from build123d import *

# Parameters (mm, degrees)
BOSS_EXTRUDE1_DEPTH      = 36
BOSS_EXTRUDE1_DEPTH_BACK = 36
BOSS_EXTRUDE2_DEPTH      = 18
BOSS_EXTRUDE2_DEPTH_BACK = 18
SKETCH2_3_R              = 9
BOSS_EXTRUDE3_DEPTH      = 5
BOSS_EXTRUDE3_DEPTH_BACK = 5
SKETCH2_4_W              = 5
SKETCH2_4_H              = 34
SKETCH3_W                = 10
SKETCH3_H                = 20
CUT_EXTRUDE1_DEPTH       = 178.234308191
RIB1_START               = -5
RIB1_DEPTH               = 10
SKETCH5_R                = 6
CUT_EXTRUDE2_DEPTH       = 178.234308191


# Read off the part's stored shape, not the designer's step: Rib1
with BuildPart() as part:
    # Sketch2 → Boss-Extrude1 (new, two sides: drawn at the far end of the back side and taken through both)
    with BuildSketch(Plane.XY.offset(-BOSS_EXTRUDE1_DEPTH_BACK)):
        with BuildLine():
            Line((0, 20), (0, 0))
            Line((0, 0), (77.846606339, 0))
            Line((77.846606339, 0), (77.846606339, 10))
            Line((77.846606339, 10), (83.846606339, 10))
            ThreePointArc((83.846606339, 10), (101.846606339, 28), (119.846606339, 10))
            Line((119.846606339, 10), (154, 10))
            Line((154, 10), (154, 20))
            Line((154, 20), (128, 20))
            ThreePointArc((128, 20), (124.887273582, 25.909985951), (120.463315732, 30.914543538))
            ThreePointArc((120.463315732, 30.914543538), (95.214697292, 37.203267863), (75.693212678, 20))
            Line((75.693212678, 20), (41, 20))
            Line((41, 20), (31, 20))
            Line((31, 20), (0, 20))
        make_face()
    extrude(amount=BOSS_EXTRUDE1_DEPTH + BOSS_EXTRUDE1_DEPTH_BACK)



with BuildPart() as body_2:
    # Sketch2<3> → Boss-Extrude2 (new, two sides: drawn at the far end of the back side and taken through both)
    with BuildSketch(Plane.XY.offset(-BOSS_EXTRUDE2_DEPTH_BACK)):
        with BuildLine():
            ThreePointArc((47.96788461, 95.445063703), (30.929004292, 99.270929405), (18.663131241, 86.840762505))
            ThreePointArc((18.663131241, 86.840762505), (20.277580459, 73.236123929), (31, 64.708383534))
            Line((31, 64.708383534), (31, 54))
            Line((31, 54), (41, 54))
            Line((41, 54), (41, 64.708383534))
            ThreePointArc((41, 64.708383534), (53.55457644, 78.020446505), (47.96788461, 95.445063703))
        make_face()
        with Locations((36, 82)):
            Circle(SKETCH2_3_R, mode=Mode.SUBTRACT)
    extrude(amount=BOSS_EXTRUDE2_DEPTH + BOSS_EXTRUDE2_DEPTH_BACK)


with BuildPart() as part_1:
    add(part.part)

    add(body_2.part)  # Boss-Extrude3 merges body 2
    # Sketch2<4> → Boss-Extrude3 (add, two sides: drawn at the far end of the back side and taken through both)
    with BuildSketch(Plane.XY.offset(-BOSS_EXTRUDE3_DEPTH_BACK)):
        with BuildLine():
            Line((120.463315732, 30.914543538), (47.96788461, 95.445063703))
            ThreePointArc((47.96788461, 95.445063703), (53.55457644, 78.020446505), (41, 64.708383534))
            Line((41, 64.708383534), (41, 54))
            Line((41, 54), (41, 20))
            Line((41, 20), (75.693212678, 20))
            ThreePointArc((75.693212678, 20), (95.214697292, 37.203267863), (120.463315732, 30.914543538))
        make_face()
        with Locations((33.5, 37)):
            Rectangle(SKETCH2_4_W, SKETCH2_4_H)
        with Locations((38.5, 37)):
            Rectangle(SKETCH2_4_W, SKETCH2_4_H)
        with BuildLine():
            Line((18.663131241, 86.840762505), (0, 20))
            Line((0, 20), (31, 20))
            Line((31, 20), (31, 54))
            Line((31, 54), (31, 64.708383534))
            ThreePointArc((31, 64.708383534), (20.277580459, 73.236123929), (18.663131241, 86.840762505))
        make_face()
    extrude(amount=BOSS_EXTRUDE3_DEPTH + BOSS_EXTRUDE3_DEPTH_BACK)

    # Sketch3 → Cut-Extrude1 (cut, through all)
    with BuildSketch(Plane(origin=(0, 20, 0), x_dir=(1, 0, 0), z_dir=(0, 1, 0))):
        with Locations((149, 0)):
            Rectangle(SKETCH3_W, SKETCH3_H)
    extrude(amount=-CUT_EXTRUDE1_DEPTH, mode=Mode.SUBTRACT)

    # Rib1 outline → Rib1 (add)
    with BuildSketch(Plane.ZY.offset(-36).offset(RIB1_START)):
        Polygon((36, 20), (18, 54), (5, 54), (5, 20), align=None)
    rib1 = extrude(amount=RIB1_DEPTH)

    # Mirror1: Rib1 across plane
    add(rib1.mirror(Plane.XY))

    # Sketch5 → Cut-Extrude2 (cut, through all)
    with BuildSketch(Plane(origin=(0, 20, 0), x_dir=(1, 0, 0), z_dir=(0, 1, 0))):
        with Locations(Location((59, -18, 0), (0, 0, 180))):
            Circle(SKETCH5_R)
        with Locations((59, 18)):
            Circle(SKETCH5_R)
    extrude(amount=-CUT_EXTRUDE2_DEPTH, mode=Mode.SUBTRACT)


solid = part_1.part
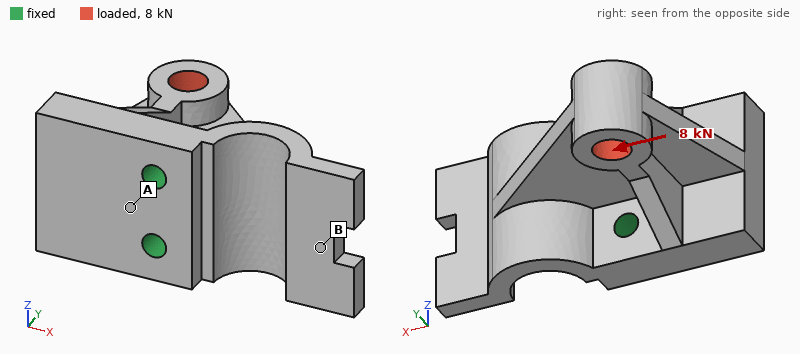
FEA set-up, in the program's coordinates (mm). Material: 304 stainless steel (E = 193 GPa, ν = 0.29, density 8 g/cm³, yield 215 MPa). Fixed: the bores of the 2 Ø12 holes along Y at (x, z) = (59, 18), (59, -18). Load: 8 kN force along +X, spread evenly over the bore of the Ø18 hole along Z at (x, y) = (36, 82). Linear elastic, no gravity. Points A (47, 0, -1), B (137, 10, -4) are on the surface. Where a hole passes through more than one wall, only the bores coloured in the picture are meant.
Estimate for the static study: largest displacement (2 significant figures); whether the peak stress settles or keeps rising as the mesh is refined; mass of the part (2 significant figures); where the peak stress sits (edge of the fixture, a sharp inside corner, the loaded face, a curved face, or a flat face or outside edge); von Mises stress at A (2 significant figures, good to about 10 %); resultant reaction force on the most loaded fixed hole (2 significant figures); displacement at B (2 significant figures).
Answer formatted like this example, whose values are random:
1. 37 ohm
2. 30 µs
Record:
1. 67 µm
2. keeps rising
3. 2.1 kg
4. edge of the fixture
5. 24 MPa
6. 4.0 kN
7. 53 µm
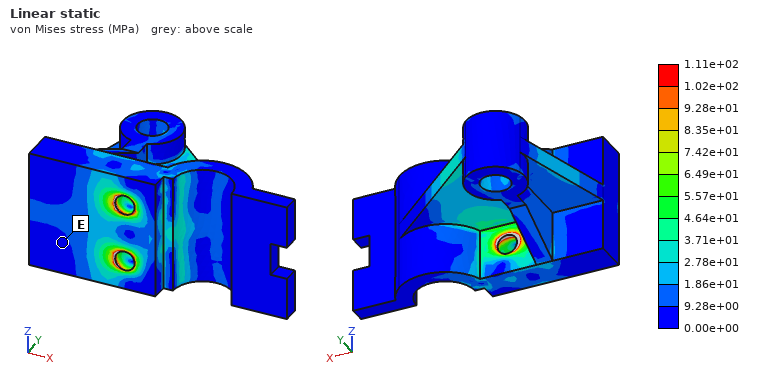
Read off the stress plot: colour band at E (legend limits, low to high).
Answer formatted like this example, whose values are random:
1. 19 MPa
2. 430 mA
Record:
1. 0.00e+00 to 9.28e+00 MPa
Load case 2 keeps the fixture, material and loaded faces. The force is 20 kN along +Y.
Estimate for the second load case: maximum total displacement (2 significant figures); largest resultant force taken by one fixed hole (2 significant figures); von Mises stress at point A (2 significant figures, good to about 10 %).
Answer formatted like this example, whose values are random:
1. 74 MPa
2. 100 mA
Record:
1. 45 µm
2. 10 kN
3. 24 MPa
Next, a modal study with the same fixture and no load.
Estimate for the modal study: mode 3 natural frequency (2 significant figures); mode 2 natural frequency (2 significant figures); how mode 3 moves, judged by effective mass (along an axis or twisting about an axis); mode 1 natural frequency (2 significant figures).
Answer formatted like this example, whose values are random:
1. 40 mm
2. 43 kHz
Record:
1. 3000 Hz
2. 2200 Hz
3. along X
4. 1700 Hz
